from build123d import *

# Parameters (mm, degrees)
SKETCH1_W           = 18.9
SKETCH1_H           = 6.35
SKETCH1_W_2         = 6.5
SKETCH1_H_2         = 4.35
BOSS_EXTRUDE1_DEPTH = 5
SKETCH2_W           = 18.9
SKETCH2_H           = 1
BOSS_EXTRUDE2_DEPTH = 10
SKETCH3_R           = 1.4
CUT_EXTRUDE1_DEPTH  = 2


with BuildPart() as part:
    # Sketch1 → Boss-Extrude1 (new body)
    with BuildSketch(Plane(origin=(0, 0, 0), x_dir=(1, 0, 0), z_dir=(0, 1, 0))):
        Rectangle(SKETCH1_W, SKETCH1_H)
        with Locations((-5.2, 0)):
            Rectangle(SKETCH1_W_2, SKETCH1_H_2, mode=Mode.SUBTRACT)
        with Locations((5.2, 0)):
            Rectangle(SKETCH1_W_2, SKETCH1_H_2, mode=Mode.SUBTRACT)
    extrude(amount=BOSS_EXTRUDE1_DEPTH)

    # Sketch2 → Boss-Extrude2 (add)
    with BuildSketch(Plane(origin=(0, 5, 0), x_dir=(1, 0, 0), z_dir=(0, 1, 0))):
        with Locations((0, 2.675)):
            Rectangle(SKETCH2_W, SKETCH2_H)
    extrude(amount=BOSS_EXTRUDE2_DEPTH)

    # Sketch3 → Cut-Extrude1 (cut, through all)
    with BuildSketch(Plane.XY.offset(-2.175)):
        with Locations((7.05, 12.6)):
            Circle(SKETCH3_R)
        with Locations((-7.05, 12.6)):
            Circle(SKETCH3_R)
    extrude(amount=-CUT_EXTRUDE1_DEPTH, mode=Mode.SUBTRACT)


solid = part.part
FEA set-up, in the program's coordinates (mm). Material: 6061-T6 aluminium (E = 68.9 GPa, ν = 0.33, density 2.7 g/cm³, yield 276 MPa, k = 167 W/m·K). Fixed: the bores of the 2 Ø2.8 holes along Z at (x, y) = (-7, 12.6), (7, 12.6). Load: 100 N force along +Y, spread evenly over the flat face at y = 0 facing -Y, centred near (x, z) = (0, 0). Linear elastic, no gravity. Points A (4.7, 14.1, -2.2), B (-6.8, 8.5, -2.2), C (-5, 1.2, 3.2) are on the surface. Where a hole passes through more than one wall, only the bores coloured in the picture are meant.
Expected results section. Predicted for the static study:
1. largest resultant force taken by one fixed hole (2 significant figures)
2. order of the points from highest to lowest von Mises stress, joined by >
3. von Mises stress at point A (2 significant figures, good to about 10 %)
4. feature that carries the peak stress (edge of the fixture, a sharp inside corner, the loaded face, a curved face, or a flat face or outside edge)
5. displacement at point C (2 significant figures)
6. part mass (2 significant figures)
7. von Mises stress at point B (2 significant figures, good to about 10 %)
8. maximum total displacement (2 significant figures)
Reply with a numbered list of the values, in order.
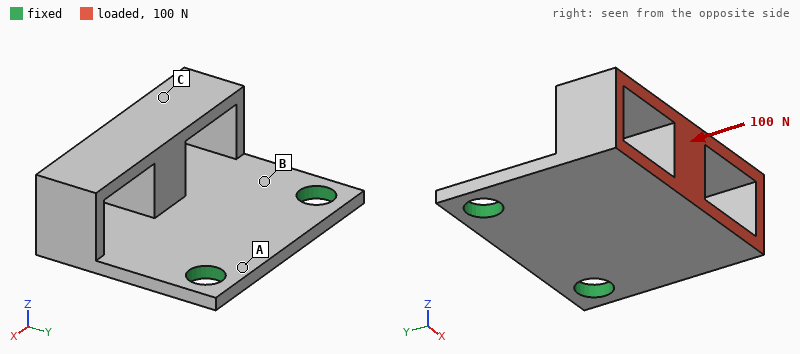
1. 52 N
2. B > A > C
3. 27 MPa
4. a flat face or outside edge
5. 0.17 mm
6. 1.3 g
7. 88 MPa
8. 0.19 mm
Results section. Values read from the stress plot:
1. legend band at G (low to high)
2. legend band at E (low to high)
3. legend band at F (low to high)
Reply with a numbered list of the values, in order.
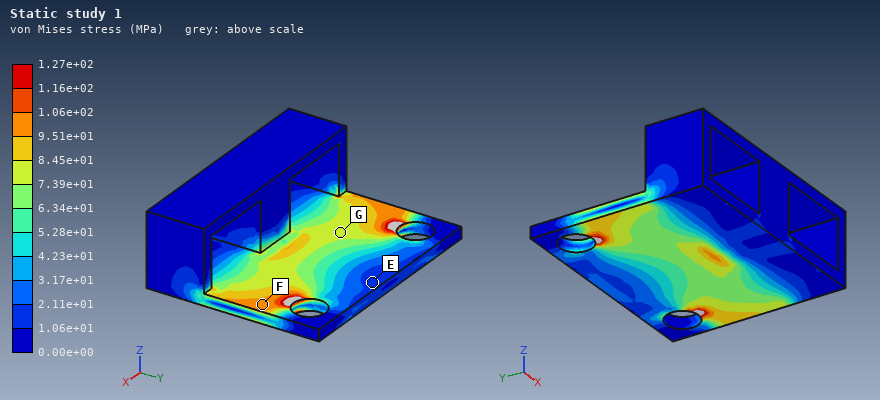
1. 7.39e+01 to 8.45e+01 MPa
2. 1.06e+01 to 2.11e+01 MPa
3. 9.51e+01 to 1.06e+02 MPa
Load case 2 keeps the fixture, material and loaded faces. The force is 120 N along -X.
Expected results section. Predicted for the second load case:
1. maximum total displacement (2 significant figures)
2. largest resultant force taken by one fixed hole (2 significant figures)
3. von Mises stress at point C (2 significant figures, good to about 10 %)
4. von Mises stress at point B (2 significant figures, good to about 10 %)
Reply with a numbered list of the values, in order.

1. 42 µm
2. 120 N
3. 9.2 MPa
4. 37 MPa
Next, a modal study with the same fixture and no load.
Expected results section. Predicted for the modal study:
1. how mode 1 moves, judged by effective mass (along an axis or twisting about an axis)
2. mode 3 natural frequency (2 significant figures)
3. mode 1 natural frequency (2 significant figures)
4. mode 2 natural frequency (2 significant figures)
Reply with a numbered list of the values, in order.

1. along Z
2. 13 kHz
3. 2900 Hz
4. 7500 Hz
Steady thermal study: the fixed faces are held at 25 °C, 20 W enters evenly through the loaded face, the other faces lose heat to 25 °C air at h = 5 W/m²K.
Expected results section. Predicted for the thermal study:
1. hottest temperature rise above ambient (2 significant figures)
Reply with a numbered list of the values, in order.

1. 78 K
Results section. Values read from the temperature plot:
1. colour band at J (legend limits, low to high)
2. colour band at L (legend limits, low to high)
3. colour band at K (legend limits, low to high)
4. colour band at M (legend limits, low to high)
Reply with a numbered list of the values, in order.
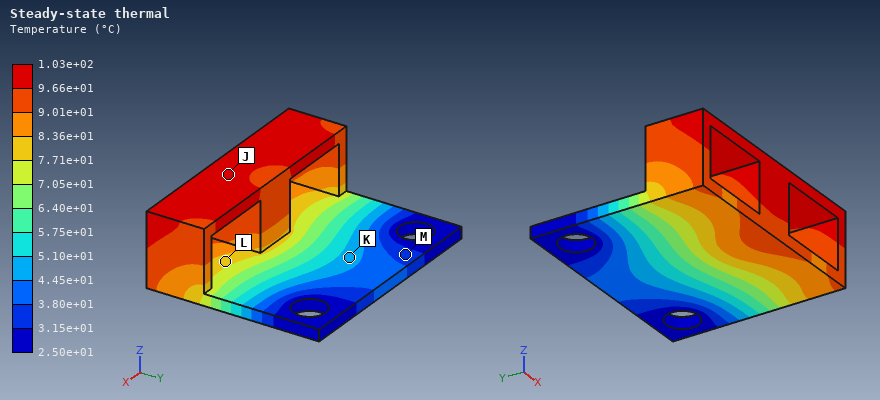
1. 9.66e+01 to 1.03e+02 °C
2. 7.71e+01 to 8.36e+01 °C
3. 4.45e+01 to 5.10e+01 °C
4. 3.15e+01 to 3.80e+01 °C
